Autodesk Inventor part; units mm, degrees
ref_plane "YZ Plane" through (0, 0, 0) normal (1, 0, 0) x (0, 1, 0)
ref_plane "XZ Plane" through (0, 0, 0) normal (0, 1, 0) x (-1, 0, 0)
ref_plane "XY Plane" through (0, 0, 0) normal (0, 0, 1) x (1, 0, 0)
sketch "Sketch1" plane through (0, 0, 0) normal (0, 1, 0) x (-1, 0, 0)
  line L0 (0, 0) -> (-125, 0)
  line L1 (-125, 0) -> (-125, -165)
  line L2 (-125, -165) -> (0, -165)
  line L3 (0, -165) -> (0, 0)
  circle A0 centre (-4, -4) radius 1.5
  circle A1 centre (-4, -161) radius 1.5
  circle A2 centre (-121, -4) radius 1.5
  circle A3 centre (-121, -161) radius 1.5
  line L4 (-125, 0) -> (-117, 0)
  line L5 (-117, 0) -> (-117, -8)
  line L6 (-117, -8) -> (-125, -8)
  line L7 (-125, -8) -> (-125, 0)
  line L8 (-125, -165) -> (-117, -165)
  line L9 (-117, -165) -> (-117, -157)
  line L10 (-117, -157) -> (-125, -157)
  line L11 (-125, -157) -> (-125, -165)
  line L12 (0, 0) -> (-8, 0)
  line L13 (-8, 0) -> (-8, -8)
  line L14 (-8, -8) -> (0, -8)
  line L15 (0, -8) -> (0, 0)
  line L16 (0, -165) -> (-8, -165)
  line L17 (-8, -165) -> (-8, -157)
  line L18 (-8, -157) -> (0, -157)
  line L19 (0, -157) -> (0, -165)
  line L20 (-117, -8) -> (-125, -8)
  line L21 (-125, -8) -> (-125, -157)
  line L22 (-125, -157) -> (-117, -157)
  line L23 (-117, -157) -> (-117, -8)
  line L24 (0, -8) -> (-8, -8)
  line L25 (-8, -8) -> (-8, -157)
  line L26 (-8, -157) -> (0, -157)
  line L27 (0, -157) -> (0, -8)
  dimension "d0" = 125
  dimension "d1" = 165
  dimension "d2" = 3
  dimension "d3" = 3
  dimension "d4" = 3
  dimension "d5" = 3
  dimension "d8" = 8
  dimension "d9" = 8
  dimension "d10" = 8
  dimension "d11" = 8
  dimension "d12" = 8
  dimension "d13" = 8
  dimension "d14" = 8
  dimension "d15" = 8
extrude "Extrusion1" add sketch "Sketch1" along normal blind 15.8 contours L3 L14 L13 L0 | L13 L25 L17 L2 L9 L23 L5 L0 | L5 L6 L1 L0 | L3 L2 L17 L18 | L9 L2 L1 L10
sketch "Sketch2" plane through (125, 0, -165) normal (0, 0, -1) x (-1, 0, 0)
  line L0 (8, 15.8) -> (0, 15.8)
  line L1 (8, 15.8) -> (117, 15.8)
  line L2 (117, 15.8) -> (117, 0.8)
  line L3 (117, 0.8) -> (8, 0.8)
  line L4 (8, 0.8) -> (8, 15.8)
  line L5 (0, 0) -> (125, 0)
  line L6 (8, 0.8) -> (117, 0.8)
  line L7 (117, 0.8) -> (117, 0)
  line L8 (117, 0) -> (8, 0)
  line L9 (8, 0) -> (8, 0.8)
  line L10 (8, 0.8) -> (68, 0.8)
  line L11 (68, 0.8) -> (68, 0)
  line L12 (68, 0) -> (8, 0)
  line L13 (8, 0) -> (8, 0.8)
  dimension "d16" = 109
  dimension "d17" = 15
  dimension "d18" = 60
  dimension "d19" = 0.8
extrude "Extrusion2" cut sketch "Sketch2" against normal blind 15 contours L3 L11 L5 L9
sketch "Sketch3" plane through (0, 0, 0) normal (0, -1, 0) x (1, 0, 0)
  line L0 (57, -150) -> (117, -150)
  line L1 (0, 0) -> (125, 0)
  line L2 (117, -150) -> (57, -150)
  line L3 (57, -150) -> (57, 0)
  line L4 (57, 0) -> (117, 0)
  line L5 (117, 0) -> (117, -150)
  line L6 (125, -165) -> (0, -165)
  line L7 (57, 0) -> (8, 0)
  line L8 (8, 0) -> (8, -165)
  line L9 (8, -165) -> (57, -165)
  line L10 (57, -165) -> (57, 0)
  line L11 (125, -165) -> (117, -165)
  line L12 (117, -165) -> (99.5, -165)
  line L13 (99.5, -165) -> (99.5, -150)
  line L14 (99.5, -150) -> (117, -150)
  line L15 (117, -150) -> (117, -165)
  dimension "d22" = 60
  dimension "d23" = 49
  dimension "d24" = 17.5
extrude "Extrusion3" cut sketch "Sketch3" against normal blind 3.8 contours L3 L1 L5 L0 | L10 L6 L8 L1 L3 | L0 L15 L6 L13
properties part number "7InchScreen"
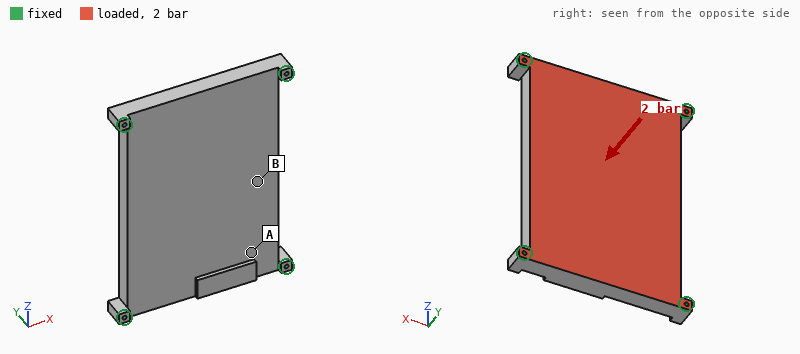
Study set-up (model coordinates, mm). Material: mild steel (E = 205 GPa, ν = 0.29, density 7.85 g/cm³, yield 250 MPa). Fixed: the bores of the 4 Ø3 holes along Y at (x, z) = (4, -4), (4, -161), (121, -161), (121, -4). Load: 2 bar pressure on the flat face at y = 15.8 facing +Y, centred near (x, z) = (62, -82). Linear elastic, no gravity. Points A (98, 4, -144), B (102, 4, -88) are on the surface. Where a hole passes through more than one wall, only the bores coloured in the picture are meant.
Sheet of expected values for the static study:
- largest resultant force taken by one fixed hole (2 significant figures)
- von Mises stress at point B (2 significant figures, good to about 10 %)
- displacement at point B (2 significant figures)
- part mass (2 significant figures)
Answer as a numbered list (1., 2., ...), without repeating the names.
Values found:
1. 920 N
2. 17 MPa
3. 36 µm
4. 1.7 kg
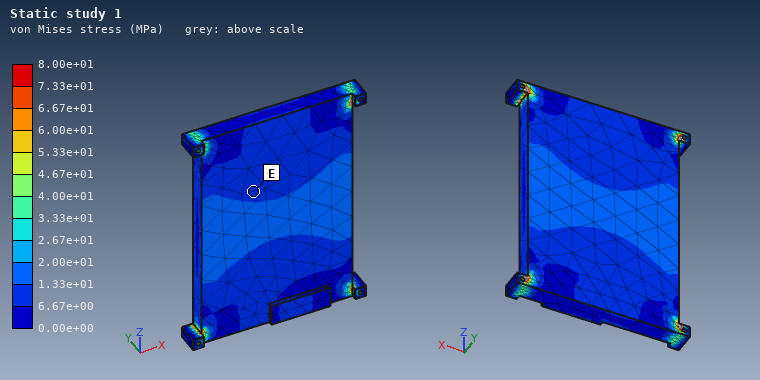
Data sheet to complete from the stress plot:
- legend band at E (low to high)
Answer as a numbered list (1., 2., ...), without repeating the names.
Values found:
1. 6.67e+00 to 1.33e+01 MPa
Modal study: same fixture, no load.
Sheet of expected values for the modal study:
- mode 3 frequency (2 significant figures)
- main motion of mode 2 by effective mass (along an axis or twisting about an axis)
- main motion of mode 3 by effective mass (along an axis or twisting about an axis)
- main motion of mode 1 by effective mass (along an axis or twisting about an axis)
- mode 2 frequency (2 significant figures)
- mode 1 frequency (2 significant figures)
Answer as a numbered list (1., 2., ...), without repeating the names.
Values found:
1. 3400 Hz
2. twisting about Z
3. twisting about X
4. along Y
5. 2700 Hz
6. 1400 Hz
